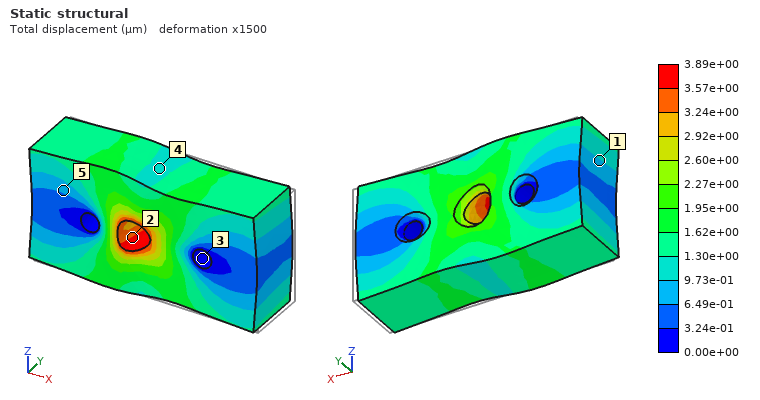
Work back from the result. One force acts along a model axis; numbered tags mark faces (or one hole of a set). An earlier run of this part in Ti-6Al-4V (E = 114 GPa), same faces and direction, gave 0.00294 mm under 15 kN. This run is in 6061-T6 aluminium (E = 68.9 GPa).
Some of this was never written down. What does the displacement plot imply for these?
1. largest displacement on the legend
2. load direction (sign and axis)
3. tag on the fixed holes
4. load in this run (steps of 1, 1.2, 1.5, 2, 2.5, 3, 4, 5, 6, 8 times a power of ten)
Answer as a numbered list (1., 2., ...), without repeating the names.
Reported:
1. 3.89e+00 µm
2. -X
3. 3
4. 12 kN
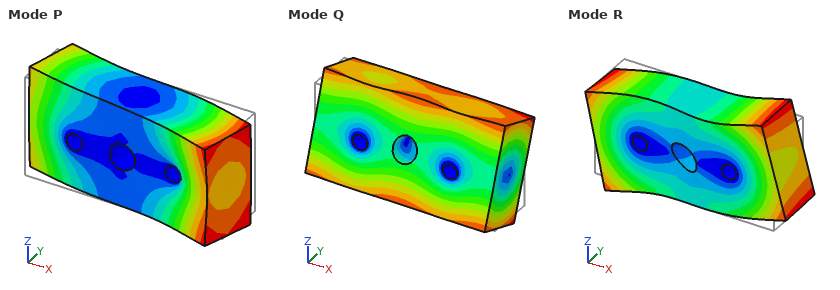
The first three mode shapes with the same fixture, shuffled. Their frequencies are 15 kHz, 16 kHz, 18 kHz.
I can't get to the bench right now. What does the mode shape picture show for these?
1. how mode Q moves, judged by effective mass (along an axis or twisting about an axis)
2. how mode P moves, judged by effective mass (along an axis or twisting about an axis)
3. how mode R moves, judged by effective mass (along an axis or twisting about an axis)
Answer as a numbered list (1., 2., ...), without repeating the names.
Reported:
1. twisting about X
2. twisting about Z
3. twisting about Y
